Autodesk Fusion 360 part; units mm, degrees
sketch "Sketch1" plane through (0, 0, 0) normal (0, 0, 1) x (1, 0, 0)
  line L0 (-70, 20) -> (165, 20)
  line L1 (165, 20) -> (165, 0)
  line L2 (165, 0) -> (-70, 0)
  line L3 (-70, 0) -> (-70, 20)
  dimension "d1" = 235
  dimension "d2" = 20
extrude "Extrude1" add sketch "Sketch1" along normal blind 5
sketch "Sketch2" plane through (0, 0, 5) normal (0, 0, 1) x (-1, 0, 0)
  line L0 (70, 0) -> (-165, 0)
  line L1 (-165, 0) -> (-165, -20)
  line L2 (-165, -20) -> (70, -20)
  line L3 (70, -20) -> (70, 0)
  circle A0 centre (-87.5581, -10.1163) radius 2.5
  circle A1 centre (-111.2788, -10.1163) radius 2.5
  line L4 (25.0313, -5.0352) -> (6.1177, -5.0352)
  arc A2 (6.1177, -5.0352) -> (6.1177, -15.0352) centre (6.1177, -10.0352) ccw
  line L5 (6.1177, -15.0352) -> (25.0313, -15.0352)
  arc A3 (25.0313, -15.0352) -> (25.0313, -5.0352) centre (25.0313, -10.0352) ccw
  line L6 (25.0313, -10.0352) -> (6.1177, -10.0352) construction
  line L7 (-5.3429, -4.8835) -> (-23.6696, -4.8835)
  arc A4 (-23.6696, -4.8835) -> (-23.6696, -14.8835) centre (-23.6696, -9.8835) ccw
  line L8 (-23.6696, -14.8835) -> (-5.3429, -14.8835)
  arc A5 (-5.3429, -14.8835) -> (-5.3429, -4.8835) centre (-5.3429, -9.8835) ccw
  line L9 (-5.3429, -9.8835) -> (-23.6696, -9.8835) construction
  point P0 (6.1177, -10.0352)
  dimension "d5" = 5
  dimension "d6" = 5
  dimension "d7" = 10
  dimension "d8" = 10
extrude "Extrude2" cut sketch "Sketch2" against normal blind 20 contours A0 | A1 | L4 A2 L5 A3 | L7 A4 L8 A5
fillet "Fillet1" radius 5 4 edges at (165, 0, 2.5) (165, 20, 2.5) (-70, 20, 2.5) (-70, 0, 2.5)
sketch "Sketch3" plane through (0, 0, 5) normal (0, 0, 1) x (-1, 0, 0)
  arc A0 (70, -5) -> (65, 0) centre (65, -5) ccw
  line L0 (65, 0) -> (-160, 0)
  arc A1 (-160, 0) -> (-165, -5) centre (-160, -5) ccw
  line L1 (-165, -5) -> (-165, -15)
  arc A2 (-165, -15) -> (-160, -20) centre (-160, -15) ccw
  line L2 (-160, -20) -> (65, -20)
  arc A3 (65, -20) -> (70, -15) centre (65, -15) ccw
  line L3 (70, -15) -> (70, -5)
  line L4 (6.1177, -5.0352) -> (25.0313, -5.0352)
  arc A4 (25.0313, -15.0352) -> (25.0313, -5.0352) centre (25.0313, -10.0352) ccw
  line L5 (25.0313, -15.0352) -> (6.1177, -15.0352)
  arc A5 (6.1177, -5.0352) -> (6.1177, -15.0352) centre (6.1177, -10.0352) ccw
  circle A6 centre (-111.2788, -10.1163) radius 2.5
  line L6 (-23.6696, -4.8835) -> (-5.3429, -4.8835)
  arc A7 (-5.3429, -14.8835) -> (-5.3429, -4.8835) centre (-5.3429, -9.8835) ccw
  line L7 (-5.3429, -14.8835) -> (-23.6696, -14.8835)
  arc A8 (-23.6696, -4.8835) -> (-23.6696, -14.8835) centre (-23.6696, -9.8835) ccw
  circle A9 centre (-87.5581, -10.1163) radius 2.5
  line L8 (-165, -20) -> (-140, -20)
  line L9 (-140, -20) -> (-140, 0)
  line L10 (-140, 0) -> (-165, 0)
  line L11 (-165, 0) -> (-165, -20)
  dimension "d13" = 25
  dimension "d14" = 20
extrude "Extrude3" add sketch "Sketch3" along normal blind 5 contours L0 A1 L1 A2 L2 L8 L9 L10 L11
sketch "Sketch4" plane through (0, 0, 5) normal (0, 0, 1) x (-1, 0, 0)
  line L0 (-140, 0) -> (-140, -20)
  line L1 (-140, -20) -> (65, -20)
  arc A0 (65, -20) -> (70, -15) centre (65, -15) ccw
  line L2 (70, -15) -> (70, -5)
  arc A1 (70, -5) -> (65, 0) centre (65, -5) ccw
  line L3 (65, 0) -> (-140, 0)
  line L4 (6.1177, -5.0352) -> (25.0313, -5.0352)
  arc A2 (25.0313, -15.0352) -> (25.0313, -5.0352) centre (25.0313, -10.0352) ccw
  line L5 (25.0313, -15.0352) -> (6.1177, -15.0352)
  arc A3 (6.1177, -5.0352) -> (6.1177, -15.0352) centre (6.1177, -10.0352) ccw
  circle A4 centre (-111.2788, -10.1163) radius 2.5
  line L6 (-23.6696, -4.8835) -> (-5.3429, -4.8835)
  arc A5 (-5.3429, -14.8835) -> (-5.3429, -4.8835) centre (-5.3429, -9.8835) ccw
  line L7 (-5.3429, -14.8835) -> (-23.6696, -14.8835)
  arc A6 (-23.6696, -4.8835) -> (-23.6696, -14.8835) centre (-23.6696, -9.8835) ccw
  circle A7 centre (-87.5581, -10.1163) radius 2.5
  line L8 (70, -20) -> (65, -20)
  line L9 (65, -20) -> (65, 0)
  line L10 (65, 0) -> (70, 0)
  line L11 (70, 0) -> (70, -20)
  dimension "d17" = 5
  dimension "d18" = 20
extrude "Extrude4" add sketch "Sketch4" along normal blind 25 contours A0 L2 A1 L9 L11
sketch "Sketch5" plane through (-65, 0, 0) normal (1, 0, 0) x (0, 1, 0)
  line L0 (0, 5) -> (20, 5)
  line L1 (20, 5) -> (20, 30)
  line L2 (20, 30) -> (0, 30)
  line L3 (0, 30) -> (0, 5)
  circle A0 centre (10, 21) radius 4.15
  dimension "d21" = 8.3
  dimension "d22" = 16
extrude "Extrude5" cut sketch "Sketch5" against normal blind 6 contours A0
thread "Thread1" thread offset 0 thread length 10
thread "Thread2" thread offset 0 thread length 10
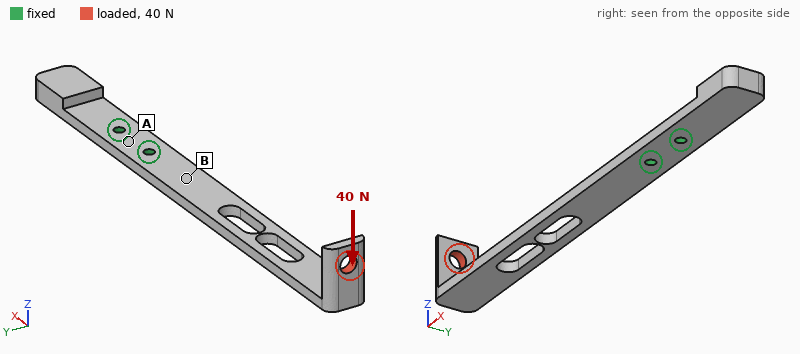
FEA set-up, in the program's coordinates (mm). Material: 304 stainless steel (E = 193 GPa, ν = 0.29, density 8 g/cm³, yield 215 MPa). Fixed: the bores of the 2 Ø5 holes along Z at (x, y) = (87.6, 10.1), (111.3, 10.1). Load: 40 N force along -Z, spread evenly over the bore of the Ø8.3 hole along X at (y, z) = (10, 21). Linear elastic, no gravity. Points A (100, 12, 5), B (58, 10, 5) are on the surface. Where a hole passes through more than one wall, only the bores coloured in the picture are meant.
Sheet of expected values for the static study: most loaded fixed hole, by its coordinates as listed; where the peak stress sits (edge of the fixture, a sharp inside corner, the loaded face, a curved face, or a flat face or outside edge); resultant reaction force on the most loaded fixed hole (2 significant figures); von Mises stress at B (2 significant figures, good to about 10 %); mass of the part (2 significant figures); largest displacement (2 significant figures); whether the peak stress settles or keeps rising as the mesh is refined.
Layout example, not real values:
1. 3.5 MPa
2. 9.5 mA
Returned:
1. (87.6, 10.1)
2. edge of the fixture
3. 82 N
4. 60 MPa
5. 200 g
6. 1.6 mm
7. keeps rising
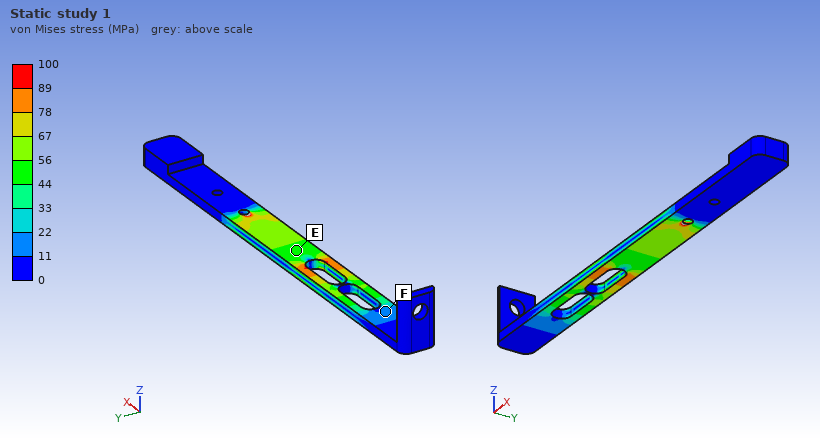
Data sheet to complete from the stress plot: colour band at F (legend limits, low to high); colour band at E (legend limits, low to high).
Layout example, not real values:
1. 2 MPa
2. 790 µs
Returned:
1. 11 to 22 MPa
2. 44 to 56 MPa
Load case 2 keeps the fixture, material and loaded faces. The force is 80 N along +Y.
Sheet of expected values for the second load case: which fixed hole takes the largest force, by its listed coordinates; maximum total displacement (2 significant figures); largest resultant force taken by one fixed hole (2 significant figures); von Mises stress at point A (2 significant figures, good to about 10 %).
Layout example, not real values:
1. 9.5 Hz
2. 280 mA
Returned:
1. (87.6, 10.1)
2. 0.43 mm
3. 410 N
4. 7.5 MPa
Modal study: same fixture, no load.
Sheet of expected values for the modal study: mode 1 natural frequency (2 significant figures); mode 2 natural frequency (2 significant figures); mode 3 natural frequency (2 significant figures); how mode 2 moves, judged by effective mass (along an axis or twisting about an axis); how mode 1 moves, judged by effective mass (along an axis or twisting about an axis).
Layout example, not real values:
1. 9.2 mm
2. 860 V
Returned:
1. 130 Hz
2. 450 Hz
3. 820 Hz
4. along Y
5. along Z
